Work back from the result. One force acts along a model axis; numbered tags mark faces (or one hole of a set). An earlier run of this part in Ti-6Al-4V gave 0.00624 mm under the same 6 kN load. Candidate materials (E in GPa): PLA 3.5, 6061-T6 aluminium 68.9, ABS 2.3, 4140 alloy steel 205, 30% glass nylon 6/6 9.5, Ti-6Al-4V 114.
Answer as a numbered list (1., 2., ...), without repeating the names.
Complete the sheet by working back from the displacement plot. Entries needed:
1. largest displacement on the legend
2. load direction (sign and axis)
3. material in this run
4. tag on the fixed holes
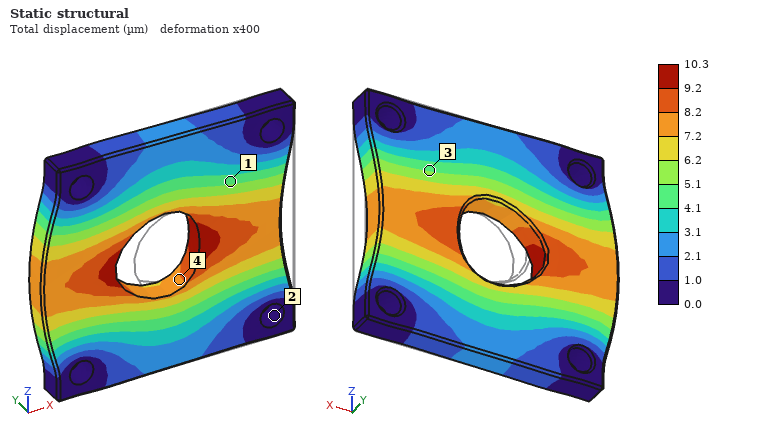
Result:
1. 10.3 µm
2. -X
3. 6061-T6 aluminium
4. 2
